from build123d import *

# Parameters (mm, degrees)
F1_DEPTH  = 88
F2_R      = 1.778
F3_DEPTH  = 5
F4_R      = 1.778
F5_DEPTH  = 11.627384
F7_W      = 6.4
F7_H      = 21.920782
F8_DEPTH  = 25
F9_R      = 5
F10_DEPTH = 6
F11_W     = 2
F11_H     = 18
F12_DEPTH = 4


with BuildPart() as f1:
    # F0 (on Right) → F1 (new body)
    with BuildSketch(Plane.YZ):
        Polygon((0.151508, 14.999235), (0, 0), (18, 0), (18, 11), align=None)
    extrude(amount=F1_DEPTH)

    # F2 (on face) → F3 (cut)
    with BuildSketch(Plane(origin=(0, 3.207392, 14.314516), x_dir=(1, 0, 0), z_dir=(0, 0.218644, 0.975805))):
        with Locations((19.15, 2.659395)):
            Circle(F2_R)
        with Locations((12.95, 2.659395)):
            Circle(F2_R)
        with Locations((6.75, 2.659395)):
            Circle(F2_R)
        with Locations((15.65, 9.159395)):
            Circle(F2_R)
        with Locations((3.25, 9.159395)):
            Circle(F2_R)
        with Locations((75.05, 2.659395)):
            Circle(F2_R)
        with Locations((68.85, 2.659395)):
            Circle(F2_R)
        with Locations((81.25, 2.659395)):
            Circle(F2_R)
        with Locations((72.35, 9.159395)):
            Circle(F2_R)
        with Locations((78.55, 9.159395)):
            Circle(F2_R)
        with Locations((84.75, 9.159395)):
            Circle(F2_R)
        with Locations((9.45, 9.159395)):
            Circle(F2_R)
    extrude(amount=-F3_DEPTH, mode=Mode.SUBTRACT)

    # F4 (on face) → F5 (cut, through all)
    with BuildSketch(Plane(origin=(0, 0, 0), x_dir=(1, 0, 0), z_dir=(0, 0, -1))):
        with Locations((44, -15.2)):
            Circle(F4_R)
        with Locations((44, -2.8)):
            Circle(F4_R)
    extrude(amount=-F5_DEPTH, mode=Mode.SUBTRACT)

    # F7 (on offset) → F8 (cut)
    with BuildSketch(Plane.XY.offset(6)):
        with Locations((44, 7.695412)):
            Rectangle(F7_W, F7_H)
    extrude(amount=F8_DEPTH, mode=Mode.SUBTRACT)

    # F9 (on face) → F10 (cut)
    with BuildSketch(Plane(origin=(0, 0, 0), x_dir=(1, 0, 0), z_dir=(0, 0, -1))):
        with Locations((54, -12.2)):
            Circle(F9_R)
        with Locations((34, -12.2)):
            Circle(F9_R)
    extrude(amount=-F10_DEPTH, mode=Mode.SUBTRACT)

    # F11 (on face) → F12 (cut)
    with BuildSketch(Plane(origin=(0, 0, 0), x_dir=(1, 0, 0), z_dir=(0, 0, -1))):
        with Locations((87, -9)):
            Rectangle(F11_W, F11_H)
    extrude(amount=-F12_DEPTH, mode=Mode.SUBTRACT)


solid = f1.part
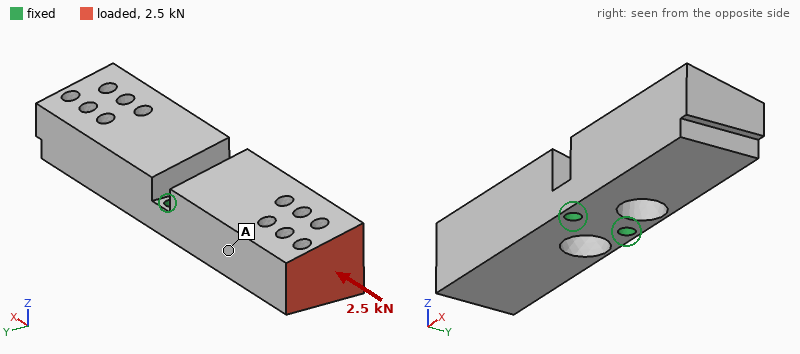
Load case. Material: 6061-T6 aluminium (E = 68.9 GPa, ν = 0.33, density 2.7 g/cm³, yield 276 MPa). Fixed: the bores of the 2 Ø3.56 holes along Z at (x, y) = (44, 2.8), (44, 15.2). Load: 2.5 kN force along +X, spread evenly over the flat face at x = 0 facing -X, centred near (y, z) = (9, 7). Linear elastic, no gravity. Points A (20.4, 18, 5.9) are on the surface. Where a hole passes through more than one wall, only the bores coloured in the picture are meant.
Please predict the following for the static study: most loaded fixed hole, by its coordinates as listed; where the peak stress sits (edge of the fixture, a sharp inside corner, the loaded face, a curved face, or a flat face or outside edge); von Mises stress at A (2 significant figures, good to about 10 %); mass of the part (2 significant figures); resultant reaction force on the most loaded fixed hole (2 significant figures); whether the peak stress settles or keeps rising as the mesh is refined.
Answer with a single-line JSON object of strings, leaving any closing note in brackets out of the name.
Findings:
{"most loaded fixed hole, by its coordinates as listed": "(44, 2.8)", "where the peak stress sits": "edge of the fixture", "von Mises stress at A": "13 MPa", "mass of the part": "48 g", "resultant reaction force on the most loaded fixed hole": "1.4 kN", "whether the peak stress settles or keeps rising as the mesh is refined": "keeps rising"}
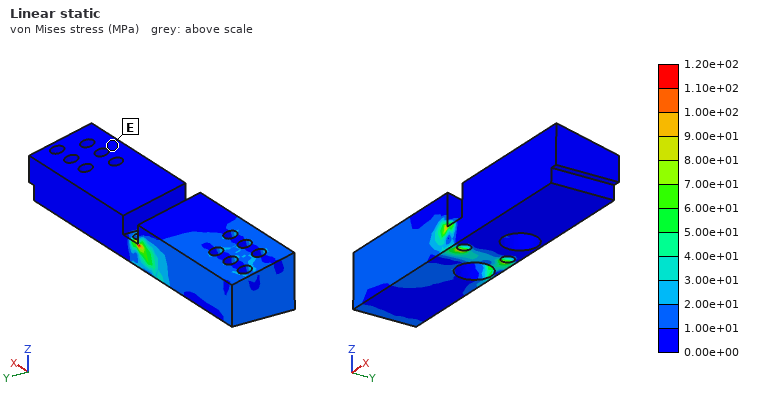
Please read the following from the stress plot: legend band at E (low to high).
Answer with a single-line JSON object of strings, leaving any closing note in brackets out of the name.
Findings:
{"legend band at E": "0.00e+00 to 1.00e+01 MPa"}
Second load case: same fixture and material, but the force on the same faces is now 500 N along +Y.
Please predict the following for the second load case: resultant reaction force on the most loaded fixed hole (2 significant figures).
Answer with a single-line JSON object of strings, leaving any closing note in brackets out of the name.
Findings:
{"resultant reaction force on the most loaded fixed hole": "1.6 kN"}
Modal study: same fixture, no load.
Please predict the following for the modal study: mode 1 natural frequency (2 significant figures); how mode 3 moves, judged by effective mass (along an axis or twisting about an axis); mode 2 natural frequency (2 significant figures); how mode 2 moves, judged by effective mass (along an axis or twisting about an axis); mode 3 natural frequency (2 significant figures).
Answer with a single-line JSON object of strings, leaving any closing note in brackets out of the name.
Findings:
{"mode 1 natural frequency": "2200 Hz", "how mode 3 moves, judged by effective mass": "along Y", "mode 2 natural frequency": "2300 Hz", "how mode 2 moves, judged by effective mass": "along Z", "mode 3 natural frequency": "4800 Hz"}
